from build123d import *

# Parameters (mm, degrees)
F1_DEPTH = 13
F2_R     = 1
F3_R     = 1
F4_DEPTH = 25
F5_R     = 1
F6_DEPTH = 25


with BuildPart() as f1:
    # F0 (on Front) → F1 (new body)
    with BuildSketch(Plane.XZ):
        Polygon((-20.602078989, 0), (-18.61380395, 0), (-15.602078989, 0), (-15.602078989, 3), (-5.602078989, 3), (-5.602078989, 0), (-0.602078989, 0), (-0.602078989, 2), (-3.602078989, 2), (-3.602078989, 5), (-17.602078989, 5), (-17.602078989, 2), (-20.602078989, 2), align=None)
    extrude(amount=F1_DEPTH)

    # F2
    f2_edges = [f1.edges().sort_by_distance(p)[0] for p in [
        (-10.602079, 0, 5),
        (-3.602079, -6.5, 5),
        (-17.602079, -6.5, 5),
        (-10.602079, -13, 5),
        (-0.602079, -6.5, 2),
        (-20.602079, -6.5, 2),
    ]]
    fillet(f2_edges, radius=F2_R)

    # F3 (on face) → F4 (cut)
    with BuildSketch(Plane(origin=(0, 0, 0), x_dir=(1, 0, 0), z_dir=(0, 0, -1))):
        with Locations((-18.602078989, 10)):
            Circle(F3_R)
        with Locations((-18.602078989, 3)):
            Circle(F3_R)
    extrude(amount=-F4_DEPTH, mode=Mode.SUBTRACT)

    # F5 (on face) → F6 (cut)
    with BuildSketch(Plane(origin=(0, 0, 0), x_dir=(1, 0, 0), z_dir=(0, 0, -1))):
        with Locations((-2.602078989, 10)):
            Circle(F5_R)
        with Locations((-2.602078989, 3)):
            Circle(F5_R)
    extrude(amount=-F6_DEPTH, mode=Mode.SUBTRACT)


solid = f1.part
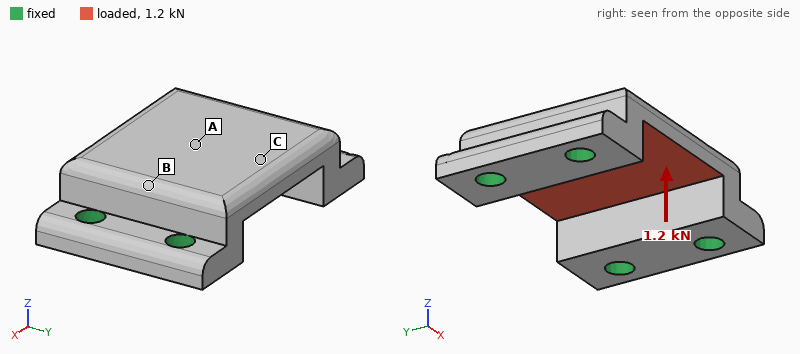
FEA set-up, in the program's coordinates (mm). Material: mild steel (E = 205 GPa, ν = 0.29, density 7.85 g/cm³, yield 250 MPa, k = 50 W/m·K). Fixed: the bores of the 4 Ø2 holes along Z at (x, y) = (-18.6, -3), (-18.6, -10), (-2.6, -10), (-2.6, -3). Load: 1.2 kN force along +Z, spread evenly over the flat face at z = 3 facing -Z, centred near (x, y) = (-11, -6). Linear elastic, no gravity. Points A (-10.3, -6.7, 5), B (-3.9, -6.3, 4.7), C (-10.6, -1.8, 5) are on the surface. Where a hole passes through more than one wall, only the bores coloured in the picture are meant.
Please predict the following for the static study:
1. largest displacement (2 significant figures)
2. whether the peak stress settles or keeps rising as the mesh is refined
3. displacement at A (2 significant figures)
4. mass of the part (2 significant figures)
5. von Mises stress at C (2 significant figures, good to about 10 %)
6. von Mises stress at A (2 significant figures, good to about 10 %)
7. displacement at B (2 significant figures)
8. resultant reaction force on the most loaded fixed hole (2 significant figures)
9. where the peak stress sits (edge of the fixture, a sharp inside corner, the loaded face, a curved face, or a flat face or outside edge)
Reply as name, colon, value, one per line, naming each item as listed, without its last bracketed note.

largest displacement: 7.1 µm
whether the peak stress settles or keeps rising as the mesh is refined: keeps rising
displacement at A: 5.9 µm
mass of the part: 5.0 g
von Mises stress at C: 120 MPa
von Mises stress at A: 110 MPa
displacement at B: 1.1 µm
resultant reaction force on the most loaded fixed hole: 430 N
where the peak stress sits: edge of the fixture
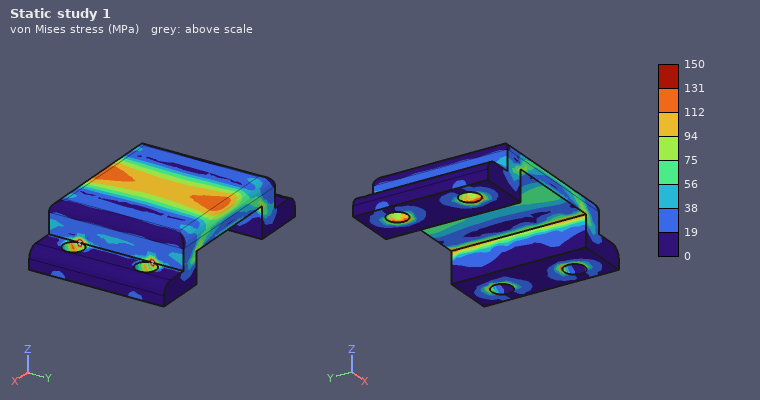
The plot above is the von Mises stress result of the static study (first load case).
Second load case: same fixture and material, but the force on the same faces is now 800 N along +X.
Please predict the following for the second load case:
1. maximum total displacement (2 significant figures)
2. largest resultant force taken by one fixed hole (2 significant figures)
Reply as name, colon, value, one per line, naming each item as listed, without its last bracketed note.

maximum total displacement: 2.4 µm
largest resultant force taken by one fixed hole: 200 N
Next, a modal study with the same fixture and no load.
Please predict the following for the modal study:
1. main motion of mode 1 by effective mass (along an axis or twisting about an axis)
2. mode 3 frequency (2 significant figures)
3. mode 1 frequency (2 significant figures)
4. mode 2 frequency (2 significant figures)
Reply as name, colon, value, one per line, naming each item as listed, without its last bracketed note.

main motion of mode 1 by effective mass: along Z
mode 3 frequency: 59 kHz
mode 1 frequency: 54 kHz
mode 2 frequency: 57 kHz
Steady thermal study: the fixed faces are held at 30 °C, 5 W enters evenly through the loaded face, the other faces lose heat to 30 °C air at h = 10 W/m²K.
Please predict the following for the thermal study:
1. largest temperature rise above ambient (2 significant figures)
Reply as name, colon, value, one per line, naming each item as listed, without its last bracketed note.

largest temperature rise above ambient: 13 K
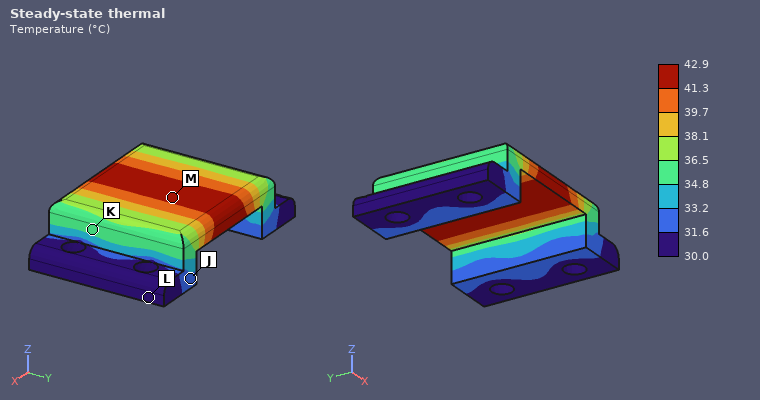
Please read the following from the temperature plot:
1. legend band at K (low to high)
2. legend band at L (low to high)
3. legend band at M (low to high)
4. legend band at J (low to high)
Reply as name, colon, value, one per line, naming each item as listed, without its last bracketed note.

legend band at K: 34.8 to 36.5 °C
legend band at L: 30.0 to 31.6 °C
legend band at M: 41.3 to 42.9 °C
legend band at J: 31.6 to 33.2 °C
